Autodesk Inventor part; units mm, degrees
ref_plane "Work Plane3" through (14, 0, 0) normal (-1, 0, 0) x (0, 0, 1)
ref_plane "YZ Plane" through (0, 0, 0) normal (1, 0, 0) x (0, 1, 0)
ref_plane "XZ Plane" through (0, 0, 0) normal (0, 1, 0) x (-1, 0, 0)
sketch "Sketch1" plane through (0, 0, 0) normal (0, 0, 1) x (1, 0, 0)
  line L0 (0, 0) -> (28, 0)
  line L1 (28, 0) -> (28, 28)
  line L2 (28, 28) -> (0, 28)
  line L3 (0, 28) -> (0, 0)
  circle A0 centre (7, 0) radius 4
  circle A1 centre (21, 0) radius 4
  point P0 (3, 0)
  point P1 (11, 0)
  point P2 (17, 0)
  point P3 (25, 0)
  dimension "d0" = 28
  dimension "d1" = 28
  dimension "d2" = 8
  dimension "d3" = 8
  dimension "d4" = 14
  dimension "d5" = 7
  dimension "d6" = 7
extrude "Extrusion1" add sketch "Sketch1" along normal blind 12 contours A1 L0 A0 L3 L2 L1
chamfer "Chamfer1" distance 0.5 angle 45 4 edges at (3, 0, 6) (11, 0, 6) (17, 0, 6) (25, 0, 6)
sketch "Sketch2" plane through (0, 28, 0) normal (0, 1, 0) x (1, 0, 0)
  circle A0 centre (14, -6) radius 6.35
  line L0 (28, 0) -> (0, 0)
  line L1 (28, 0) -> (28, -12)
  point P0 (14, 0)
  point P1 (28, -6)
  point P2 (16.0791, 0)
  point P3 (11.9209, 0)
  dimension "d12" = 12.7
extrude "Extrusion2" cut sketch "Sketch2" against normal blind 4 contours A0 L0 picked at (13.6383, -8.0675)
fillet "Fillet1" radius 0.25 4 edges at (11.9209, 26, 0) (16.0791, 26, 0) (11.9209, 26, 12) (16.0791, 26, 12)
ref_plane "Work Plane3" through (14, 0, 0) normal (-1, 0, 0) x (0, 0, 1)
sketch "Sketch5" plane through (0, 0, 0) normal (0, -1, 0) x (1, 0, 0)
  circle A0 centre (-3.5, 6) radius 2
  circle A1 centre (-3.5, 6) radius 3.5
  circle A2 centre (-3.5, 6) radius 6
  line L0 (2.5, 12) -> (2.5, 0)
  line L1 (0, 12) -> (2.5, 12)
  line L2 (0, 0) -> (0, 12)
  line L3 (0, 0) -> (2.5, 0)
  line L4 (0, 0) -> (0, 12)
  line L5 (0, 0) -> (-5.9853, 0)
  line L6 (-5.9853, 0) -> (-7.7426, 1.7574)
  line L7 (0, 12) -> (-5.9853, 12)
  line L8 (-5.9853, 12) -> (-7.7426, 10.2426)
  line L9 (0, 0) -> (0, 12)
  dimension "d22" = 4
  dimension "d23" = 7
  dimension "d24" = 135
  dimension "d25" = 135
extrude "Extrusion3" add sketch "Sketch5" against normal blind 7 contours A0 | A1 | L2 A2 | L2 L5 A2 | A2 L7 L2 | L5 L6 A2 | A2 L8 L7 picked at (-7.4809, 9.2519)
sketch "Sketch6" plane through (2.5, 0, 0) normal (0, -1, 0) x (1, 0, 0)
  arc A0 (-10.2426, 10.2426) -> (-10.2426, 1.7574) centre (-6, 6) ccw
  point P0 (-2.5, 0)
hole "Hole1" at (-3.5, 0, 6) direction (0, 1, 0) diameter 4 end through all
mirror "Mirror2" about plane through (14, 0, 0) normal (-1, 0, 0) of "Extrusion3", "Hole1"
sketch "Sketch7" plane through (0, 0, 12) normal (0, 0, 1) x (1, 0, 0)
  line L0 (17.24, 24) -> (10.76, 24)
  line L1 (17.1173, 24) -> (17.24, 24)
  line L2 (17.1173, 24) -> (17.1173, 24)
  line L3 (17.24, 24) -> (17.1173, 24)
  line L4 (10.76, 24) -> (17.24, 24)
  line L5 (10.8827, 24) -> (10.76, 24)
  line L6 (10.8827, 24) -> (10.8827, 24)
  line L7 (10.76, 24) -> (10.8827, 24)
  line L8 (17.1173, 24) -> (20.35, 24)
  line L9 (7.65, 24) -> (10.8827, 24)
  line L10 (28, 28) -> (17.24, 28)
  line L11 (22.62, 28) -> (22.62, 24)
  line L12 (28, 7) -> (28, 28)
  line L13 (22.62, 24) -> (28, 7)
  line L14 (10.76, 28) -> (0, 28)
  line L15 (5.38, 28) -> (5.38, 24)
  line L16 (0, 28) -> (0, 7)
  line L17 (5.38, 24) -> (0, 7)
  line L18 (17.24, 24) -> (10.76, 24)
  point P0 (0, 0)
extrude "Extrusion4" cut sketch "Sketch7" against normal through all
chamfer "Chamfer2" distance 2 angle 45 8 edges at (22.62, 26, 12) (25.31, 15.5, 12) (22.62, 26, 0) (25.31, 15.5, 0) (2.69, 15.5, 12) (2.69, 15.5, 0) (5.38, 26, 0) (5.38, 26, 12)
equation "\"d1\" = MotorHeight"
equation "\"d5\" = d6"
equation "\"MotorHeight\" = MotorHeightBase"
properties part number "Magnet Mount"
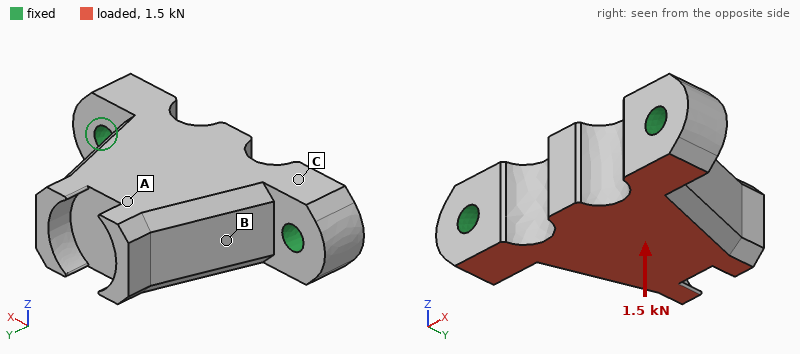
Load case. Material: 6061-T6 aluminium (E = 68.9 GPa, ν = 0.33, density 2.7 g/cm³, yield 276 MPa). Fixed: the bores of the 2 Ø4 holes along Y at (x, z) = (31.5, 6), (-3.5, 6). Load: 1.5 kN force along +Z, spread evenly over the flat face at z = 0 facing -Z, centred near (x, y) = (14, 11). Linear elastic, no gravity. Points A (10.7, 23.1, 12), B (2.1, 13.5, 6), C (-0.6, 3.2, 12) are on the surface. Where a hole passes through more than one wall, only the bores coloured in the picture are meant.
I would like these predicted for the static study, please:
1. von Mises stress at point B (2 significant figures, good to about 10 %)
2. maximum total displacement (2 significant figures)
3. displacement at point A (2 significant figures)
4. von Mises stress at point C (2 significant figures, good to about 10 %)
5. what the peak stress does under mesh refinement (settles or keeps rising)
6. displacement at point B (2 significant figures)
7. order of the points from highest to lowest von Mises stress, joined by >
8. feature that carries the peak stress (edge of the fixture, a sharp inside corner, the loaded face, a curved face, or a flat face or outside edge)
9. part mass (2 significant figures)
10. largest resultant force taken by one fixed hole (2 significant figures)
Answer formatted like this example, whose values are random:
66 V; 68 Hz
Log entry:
18 MPa; 50 µm; 39 µm; 41 MPa; keeps rising; 19 µm; C > B > A; edge of the fixture; 21 g; 750 N
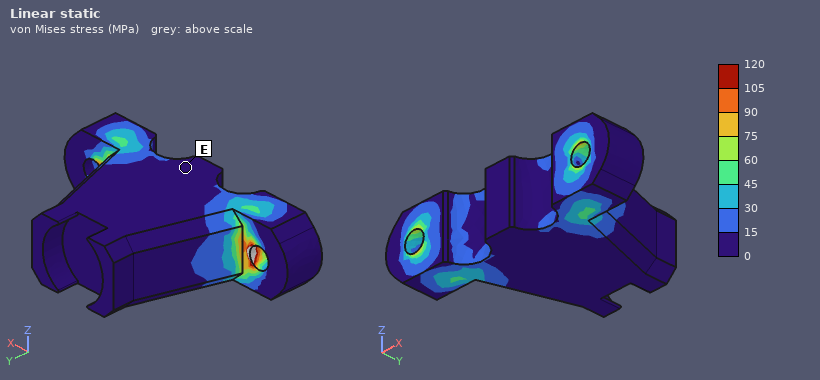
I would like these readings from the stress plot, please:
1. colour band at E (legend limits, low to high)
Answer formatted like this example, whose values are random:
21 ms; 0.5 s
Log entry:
0 to 15 MPa
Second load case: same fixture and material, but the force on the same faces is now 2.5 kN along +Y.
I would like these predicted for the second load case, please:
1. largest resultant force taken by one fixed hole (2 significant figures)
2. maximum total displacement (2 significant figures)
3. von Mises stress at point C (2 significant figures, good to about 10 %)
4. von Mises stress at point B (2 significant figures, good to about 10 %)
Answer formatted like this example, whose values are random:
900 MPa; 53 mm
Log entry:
1.4 kN; 59 µm; 34 MPa; 18 MPa
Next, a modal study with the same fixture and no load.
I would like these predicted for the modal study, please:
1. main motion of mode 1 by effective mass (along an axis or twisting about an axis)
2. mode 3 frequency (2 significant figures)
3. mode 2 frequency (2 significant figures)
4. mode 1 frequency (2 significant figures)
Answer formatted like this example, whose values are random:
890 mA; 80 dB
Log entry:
along Z; 24 kHz; 23 kHz; 7800 Hz
